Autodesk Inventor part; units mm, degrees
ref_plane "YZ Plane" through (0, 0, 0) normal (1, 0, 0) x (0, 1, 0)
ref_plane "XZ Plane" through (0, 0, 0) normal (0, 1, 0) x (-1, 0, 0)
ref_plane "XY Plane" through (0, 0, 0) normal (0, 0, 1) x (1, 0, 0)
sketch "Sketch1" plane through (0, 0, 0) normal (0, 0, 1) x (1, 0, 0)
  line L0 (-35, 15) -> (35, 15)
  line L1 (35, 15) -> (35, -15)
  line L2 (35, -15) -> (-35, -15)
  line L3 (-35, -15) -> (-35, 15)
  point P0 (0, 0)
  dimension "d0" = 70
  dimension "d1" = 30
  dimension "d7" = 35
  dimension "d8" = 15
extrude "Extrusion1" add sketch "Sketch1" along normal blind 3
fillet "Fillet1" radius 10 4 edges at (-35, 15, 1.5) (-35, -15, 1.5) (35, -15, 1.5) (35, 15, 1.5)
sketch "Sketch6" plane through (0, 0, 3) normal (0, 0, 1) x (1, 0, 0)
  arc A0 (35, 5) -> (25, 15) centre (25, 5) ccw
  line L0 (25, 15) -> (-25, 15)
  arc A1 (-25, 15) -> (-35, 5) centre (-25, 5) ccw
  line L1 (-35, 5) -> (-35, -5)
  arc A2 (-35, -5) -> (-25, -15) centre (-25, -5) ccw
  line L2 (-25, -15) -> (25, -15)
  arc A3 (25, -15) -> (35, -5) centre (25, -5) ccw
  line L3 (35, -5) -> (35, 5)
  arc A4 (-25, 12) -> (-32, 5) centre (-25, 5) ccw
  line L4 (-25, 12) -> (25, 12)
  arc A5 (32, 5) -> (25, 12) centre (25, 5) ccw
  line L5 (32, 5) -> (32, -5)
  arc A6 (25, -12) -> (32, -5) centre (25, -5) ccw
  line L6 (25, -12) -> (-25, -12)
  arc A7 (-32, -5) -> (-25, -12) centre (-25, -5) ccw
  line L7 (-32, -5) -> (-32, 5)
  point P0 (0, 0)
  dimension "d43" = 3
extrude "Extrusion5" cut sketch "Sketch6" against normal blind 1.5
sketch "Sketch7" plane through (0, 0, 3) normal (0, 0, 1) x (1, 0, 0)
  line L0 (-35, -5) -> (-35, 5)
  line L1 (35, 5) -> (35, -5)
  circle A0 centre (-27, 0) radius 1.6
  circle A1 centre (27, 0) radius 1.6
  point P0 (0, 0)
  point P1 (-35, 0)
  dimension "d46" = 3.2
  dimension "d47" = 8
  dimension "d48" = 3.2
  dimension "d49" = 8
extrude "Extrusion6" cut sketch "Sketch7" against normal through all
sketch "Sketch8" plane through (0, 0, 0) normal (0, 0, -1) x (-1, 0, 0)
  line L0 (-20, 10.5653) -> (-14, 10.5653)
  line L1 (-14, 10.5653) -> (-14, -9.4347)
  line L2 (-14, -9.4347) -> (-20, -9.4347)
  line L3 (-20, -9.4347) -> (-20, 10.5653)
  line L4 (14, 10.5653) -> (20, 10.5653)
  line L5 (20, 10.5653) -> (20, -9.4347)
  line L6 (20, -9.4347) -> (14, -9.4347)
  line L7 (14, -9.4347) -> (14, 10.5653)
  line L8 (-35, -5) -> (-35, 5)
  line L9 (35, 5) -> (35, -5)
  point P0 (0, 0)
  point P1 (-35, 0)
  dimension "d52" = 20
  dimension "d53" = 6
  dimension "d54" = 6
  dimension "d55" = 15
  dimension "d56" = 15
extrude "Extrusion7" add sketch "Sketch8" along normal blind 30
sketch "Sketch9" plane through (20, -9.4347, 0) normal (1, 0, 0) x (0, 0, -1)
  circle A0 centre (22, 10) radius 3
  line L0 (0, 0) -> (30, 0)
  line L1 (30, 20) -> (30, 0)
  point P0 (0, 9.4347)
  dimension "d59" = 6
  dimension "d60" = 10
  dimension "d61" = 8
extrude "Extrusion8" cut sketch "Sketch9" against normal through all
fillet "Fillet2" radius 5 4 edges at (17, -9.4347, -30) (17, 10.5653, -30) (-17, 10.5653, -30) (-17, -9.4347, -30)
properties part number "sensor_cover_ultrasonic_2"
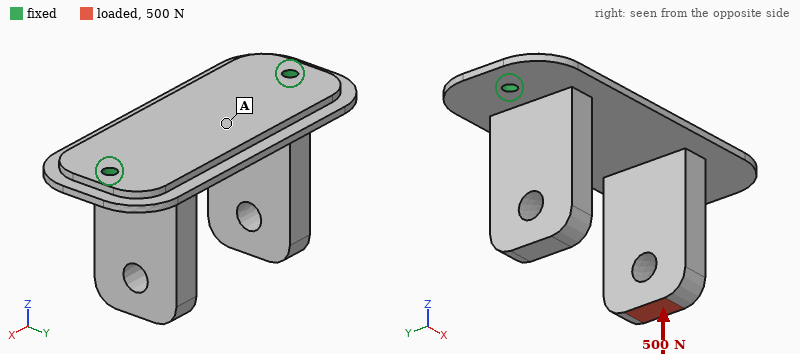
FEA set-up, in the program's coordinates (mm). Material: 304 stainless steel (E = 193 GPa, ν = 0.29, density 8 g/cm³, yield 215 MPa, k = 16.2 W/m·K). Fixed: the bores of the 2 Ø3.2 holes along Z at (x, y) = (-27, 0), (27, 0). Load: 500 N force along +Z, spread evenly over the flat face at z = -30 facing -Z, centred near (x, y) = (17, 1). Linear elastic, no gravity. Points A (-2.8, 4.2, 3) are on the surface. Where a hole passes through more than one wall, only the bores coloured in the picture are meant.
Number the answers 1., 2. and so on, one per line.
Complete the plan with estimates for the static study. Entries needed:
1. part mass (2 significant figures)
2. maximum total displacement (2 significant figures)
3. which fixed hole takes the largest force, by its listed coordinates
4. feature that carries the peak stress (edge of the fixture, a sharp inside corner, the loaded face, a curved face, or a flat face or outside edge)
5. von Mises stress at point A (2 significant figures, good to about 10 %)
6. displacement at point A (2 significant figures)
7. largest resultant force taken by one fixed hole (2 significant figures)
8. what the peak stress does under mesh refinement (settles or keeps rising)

1. 96 g
2. 36 µm
3. (27, 0)
4. edge of the fixture
5. 11 MPa
6. 14 µm
7. 440 N
8. keeps rising
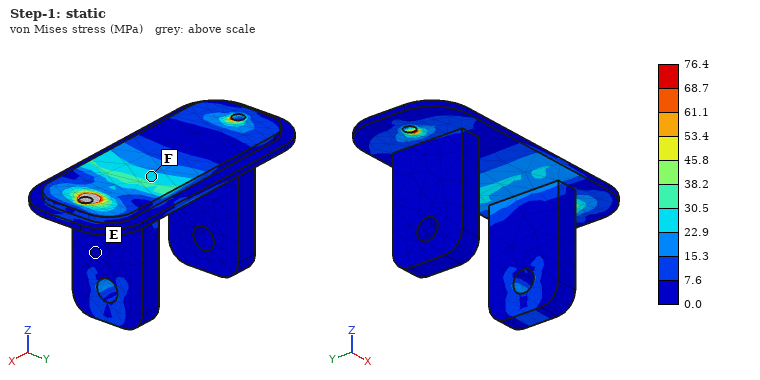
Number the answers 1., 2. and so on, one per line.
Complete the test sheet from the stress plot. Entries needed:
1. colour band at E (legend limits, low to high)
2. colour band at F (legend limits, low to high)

1. 0.0 to 7.6 MPa
2. 22.9 to 30.5 MPa
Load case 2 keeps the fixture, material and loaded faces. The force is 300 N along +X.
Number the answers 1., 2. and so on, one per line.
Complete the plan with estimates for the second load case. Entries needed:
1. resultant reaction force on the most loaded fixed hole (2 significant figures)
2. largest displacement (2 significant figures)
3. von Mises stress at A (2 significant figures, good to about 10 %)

1. 230 N
2. 0.15 mm
3. 34 MPa
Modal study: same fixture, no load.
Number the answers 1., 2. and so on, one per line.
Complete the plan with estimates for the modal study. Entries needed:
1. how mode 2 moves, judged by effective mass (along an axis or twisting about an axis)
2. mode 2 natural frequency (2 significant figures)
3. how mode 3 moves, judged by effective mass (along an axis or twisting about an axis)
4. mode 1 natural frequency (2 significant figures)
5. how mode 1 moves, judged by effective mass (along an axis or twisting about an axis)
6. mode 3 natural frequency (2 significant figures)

1. along Y
2. 2200 Hz
3. twisting about Z
4. 1900 Hz
5. along Z
6. 3000 Hz
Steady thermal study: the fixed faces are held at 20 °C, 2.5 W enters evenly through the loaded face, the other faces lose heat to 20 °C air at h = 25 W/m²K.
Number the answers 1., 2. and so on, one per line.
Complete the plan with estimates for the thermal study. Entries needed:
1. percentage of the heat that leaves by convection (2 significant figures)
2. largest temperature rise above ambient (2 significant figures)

1. 58 %
2. 48 K
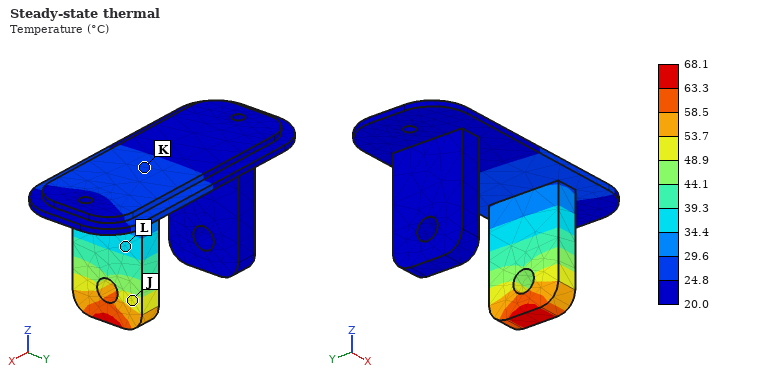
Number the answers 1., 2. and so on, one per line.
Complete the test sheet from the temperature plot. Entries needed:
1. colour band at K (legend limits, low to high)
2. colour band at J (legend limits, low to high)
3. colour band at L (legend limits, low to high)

1. 24.8 to 29.6 °C
2. 48.9 to 53.7 °C
3. 34.4 to 39.3 °C
